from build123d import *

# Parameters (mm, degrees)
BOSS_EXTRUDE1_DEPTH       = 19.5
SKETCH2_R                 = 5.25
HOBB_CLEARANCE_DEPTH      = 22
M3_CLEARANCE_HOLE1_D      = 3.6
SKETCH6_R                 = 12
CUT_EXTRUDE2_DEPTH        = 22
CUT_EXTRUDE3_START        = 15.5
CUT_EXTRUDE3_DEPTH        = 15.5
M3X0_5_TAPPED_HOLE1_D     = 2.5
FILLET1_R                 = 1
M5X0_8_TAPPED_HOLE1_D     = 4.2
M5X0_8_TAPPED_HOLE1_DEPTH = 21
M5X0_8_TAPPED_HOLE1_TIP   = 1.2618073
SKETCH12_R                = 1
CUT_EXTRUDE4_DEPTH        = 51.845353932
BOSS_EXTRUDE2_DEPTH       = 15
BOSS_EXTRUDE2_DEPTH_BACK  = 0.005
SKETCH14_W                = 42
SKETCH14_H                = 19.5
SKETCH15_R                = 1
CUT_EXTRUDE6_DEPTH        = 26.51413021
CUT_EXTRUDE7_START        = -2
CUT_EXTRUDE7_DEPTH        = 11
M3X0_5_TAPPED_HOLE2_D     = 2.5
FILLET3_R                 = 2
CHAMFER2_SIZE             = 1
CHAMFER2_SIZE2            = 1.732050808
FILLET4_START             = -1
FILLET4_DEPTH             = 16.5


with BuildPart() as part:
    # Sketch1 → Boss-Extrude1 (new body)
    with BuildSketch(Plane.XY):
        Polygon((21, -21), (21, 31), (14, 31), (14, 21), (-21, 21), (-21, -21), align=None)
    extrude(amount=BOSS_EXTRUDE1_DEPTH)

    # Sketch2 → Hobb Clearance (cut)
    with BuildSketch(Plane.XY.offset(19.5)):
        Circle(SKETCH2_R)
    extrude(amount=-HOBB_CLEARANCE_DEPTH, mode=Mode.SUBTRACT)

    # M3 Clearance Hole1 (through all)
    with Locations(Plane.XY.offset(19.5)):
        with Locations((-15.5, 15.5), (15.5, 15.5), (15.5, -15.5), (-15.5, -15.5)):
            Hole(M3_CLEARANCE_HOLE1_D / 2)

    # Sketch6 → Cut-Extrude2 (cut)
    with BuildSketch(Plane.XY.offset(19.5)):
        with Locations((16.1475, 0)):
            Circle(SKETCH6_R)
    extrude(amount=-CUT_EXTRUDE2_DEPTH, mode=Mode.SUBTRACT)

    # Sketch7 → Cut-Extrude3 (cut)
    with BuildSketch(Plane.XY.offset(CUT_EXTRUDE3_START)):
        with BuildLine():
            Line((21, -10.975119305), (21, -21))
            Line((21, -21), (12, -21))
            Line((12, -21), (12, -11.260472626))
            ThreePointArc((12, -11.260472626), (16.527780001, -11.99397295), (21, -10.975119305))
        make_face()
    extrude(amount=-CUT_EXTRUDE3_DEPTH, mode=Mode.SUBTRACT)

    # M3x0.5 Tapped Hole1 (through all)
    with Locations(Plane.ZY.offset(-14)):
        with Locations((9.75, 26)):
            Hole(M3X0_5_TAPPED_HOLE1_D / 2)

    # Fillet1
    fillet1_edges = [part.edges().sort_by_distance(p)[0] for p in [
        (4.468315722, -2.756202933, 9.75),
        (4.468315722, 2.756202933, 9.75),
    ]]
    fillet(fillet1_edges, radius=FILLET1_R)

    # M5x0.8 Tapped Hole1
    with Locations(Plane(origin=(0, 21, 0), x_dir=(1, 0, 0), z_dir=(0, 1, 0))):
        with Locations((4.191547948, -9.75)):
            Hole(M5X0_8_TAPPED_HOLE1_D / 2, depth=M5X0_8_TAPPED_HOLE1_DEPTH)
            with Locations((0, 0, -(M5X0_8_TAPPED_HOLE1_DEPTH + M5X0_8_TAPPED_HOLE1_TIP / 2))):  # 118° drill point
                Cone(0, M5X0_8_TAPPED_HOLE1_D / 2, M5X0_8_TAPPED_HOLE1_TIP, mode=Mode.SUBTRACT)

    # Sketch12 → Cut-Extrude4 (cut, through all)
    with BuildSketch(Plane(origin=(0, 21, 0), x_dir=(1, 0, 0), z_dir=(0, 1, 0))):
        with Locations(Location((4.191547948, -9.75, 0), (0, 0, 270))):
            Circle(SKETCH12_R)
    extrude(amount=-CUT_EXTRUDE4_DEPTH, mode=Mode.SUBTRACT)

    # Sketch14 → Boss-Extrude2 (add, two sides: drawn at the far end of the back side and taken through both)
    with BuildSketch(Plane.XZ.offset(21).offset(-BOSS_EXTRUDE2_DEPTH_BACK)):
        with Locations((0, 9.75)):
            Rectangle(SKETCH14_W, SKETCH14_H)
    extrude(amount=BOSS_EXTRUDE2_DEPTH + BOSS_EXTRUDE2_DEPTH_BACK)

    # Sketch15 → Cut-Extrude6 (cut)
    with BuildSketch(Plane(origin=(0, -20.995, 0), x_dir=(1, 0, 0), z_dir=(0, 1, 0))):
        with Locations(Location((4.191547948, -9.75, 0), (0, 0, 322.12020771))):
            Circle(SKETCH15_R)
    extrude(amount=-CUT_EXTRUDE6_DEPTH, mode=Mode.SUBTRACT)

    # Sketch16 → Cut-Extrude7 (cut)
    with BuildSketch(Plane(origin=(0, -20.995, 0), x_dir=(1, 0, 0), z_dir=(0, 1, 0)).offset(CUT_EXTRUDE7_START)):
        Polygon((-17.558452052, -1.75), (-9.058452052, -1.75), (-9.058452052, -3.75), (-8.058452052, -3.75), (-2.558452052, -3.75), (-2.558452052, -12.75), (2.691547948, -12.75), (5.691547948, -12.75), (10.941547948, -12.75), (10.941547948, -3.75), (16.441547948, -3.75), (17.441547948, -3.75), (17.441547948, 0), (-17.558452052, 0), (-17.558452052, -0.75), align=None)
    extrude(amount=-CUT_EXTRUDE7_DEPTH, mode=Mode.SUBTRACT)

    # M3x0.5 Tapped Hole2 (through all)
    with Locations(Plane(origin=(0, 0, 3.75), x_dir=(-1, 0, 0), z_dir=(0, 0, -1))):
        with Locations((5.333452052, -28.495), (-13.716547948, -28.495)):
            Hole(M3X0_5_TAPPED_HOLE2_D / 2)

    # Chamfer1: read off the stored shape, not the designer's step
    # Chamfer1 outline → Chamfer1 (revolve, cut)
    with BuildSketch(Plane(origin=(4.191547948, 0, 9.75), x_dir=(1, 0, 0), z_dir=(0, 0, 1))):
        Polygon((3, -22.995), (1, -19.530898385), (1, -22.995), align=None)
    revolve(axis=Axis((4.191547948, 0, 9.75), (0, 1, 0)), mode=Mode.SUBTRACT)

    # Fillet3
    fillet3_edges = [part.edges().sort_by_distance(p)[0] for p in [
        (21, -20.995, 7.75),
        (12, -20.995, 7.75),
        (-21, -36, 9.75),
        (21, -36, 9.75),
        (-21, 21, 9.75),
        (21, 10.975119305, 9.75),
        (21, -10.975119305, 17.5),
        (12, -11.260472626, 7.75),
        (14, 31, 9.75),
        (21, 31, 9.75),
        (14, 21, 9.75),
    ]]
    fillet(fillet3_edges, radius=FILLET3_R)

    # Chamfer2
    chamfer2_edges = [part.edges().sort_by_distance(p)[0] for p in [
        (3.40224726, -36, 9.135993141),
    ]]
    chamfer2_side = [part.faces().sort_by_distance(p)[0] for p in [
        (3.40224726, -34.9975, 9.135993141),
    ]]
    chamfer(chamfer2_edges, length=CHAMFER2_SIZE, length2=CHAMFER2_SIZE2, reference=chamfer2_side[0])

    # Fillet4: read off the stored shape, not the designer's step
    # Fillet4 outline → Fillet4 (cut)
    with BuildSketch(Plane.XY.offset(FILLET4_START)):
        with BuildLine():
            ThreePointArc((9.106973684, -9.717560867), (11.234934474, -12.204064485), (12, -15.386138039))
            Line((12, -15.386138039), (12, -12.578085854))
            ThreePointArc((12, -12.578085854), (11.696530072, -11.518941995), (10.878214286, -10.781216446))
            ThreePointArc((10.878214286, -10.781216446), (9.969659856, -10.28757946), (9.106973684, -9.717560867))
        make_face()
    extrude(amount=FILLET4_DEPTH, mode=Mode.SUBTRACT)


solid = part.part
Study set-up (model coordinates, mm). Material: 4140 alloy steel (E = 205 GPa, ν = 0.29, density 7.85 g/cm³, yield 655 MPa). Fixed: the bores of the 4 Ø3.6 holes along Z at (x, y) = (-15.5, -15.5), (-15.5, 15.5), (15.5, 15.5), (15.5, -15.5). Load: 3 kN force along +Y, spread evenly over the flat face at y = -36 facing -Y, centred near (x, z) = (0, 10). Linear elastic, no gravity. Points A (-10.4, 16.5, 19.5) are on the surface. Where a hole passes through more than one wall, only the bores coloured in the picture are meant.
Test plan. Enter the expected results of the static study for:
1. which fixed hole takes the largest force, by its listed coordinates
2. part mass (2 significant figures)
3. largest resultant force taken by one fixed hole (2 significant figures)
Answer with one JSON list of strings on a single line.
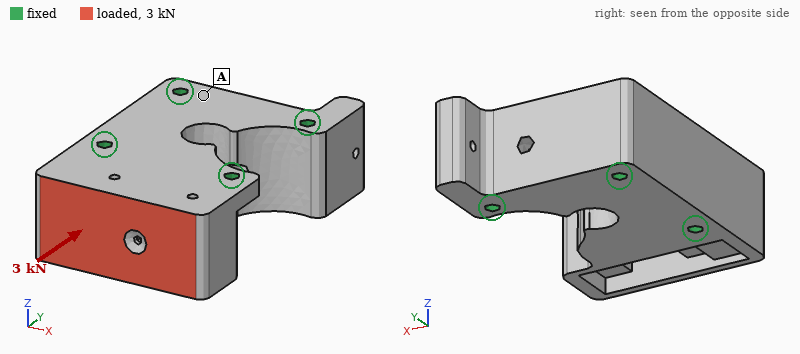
["(-15.5, -15.5)", "270 g", "1.5 kN"]
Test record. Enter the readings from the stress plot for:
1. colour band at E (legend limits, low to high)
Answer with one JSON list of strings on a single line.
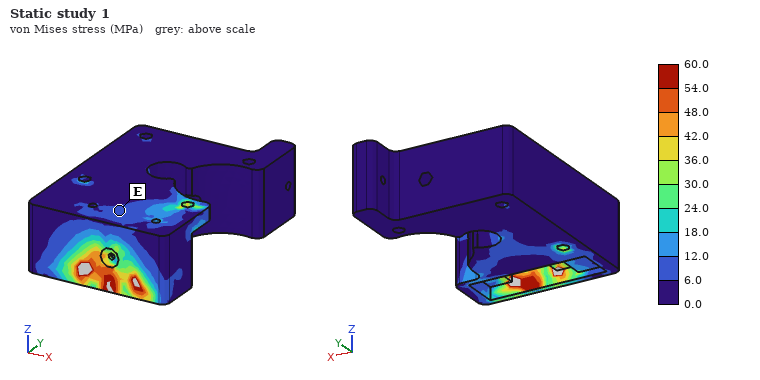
["6.0 to 12.0 MPa"]
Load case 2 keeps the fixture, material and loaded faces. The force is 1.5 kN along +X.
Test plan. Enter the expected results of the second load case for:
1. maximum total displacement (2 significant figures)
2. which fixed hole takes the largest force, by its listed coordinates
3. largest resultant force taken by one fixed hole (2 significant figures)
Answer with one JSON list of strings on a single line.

["3.3 µm", "(-15.5, -15.5)", "1.6 kN"]
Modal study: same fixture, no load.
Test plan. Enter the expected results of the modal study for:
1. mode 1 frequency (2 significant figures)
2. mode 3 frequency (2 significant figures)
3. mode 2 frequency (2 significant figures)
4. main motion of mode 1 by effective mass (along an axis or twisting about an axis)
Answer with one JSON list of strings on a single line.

["13 kHz", "25 kHz", "20 kHz", "along Z"]
